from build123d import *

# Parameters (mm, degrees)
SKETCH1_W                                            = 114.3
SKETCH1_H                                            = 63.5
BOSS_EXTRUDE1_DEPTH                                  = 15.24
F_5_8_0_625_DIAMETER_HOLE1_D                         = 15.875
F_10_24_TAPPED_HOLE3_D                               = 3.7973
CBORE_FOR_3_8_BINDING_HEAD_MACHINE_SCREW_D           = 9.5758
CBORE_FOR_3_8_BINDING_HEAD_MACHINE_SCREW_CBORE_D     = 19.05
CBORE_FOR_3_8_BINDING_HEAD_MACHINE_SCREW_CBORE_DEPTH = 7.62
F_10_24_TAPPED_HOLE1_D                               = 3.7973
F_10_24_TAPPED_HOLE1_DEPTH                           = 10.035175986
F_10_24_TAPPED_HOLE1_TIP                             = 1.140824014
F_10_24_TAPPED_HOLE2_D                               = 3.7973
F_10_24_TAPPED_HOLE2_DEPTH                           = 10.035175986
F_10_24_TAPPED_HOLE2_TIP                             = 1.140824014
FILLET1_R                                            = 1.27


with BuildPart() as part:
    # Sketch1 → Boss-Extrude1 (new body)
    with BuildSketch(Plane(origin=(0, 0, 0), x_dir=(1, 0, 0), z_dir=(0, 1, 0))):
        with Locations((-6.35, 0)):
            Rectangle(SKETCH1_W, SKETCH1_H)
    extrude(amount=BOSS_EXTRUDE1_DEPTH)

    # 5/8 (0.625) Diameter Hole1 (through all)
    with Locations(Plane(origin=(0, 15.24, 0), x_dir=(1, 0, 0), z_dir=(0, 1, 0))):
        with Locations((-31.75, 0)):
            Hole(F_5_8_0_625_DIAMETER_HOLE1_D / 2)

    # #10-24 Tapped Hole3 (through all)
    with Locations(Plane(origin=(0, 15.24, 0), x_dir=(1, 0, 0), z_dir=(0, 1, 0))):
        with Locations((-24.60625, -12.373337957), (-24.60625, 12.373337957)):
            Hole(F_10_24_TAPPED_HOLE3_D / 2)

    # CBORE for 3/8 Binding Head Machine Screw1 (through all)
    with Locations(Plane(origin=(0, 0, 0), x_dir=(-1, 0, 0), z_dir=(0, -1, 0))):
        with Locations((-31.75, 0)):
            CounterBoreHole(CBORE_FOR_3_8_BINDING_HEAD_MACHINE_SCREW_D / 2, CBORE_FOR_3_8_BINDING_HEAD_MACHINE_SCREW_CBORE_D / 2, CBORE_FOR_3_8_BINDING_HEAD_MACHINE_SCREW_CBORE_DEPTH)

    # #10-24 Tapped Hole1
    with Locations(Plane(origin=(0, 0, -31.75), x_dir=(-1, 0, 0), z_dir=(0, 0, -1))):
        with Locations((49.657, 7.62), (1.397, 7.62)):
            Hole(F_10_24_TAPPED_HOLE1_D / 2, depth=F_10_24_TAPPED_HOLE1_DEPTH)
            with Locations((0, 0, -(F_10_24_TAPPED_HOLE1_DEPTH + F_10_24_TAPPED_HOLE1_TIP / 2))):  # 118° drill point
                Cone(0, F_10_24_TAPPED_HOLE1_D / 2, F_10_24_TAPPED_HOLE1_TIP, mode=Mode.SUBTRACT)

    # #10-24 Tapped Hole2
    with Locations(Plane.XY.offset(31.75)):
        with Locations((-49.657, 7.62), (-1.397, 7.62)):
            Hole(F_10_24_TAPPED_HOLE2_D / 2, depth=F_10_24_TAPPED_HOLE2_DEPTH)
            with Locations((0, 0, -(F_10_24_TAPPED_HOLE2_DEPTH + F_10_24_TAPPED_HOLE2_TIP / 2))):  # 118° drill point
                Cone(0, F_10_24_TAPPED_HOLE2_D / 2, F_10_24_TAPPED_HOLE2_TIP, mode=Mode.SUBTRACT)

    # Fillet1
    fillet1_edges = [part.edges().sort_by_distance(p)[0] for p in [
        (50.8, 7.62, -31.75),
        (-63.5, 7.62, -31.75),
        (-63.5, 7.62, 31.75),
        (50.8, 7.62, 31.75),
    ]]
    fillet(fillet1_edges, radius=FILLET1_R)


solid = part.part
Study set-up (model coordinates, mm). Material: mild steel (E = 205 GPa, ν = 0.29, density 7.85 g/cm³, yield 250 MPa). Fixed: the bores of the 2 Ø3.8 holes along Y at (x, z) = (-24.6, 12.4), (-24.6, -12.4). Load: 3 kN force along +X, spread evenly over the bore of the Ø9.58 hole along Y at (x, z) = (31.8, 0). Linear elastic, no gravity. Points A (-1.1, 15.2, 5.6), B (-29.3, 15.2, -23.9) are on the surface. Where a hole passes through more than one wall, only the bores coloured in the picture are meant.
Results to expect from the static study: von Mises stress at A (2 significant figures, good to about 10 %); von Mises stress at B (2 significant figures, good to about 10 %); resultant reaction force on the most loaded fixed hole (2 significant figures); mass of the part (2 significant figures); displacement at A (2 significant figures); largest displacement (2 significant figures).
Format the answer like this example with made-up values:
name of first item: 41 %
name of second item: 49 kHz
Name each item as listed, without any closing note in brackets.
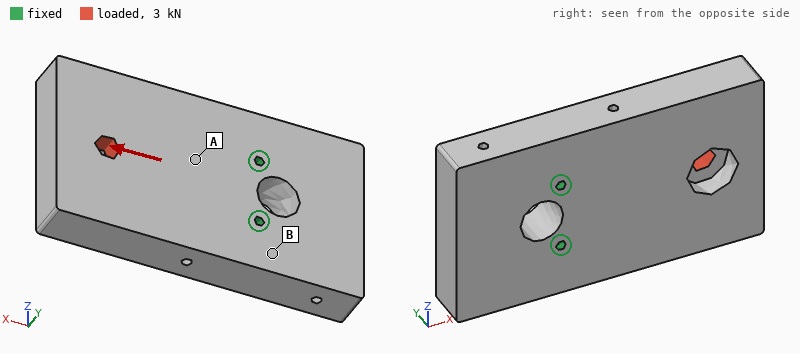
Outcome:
von Mises stress at A: 8.5 MPa
von Mises stress at B: 3.1 MPa
resultant reaction force on the most loaded fixed hole: 1.5 kN
mass of the part: 820 g
displacement at A: 1.9 µm
largest displacement: 9.8 µm
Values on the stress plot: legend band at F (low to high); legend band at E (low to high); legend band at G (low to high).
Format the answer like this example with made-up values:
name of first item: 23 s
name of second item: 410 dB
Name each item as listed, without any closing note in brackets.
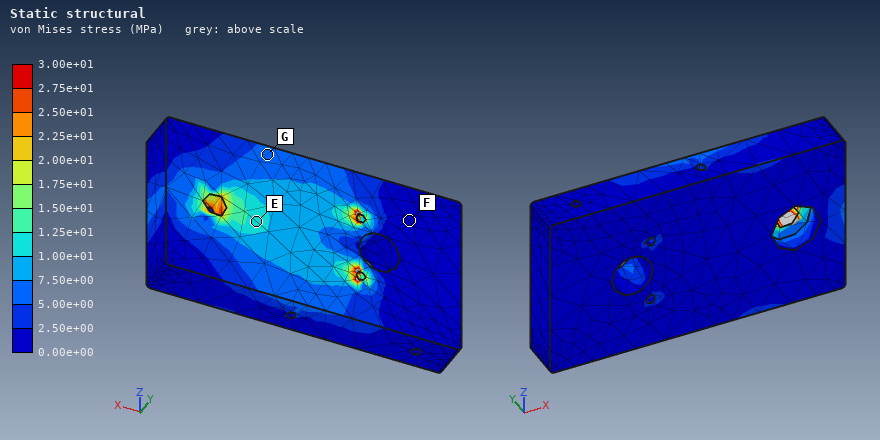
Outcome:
legend band at F: 0.00e+00 to 2.50e+00 MPa
legend band at E: 1.00e+01 to 1.25e+01 MPa
legend band at G: 5.00e+00 to 7.50e+00 MPa
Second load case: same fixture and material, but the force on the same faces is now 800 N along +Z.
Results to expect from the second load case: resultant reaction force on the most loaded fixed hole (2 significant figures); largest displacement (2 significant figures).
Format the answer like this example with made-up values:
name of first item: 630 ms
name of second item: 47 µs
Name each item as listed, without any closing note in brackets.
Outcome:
resultant reaction force on the most loaded fixed hole: 1.7 kN
largest displacement: 4.5 µm
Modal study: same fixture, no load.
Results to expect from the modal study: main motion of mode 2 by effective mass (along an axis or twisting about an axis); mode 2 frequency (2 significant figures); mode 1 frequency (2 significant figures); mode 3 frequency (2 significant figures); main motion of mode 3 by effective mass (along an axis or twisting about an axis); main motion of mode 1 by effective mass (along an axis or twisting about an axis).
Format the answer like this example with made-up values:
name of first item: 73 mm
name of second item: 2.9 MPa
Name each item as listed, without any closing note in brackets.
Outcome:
main motion of mode 2 by effective mass: along Z
mode 2 frequency: 4200 Hz
mode 1 frequency: 1900 Hz
mode 3 frequency: 4700 Hz
main motion of mode 3 by effective mass: twisting about X
main motion of mode 1 by effective mass: along Y
